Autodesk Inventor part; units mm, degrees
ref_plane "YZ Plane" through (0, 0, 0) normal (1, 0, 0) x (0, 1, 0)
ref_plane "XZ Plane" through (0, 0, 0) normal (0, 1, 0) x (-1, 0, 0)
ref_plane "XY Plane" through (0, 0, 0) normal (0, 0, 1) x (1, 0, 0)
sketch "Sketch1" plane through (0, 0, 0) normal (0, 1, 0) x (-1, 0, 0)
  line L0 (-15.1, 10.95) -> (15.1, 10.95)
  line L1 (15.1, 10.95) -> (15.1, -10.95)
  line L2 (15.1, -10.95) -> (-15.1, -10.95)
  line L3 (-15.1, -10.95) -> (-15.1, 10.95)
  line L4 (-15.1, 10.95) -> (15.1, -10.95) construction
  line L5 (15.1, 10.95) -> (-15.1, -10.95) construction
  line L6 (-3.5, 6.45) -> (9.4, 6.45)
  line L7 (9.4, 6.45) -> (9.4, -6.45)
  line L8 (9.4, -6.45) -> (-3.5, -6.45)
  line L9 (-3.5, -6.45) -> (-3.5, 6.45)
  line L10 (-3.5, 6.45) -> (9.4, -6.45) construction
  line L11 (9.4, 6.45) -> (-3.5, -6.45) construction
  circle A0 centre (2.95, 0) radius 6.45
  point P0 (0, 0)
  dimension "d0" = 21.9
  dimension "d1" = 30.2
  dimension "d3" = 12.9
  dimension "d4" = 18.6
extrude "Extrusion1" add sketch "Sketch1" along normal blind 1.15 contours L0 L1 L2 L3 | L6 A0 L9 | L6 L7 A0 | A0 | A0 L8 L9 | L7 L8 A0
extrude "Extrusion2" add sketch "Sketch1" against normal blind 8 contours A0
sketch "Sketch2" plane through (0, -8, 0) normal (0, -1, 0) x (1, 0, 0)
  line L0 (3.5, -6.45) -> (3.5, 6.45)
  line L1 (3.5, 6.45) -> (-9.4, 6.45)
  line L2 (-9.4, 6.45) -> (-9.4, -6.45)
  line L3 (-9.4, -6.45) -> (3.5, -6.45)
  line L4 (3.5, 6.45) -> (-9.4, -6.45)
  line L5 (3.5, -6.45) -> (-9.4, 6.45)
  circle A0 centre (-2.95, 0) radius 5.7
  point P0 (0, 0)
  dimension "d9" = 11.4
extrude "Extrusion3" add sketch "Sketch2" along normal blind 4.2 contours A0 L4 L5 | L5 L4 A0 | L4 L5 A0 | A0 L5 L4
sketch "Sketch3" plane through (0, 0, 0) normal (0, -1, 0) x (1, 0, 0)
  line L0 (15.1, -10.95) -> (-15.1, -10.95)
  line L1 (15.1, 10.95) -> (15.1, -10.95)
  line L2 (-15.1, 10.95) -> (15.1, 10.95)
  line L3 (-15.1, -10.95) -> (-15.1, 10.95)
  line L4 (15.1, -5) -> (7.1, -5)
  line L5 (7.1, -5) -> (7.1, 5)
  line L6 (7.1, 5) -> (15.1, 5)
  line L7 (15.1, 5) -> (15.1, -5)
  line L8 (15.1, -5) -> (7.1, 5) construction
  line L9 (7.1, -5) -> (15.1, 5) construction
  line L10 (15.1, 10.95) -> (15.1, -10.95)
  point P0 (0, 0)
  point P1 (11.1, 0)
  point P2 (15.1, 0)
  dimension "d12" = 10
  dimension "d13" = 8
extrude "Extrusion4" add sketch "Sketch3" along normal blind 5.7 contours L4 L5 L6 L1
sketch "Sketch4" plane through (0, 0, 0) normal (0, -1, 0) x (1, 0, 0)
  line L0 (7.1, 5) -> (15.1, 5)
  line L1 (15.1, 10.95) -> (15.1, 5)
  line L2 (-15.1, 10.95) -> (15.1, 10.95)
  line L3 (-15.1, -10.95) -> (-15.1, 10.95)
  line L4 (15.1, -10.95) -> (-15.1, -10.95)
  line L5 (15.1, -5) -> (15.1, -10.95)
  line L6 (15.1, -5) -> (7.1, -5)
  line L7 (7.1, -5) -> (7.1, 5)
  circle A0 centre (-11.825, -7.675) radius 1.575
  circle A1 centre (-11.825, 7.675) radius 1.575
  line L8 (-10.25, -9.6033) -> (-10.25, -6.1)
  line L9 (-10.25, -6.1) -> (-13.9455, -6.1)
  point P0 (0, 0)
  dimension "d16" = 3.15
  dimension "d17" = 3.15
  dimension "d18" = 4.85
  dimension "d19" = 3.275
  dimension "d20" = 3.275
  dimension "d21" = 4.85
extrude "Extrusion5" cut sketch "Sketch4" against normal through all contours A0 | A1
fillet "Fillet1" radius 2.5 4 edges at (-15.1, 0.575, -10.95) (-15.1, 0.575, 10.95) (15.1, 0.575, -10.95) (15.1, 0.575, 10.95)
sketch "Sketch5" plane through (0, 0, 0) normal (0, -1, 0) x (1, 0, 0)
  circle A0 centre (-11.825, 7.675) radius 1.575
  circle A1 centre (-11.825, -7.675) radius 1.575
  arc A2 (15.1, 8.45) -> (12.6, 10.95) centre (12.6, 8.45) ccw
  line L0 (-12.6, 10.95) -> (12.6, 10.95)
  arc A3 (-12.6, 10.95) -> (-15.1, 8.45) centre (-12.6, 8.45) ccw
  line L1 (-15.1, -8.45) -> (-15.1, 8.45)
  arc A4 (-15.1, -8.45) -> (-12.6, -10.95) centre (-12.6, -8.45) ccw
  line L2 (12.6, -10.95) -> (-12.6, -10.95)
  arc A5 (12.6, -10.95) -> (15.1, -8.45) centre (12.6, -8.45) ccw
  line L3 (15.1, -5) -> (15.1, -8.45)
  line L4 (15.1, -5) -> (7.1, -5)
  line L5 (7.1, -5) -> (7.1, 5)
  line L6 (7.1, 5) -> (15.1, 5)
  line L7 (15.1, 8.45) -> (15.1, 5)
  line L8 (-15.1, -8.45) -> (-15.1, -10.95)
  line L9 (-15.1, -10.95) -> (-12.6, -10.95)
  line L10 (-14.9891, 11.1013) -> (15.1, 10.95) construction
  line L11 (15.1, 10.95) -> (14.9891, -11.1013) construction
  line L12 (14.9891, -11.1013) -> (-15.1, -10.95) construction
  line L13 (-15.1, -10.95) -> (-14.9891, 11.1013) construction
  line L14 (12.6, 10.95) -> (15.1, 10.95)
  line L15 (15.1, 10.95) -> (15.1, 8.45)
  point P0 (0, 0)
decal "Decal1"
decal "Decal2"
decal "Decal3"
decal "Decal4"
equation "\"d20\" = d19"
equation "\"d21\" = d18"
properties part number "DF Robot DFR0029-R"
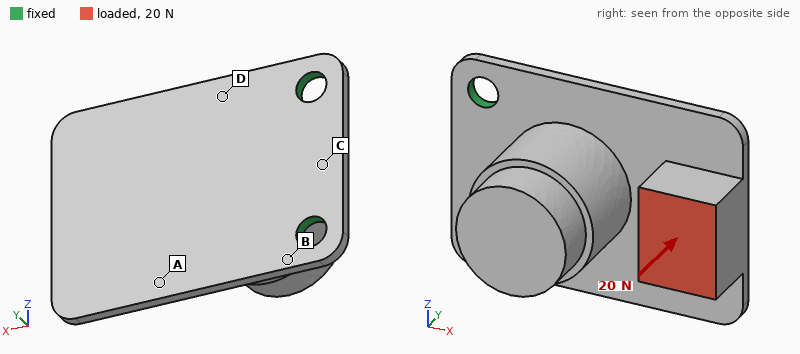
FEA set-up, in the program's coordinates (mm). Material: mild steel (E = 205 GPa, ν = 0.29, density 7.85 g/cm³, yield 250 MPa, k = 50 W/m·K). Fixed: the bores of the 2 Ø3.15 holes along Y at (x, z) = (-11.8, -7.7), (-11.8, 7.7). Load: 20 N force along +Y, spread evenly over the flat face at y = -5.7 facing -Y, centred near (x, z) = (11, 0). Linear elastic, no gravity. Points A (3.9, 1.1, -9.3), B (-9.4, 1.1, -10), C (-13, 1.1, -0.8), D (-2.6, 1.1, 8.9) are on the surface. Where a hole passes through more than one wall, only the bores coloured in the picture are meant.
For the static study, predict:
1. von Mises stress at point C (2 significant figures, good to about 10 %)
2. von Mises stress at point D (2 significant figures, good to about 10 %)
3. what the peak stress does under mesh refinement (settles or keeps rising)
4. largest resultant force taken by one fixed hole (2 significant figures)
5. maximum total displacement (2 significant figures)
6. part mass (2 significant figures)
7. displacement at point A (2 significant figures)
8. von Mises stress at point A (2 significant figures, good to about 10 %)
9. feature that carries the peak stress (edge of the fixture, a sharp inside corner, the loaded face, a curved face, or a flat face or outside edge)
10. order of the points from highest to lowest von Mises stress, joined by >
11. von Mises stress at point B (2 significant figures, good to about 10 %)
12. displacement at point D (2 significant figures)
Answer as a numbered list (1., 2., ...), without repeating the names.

1. 27 MPa
2. 8.9 MPa
3. keeps rising
4. 10 N
5. 77 µm
6. 21 g
7. 33 µm
8. 18 MPa
9. edge of the fixture
10. B > C > A > D
11. 67 MPa
12. 16 µm
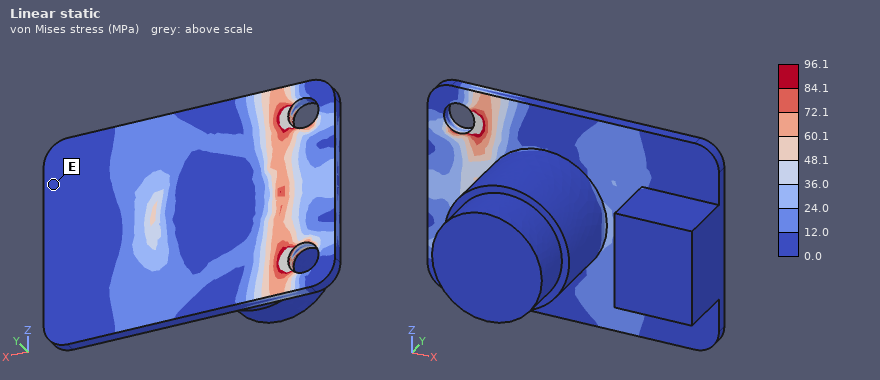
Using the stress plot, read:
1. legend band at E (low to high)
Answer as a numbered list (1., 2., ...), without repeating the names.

1. 0.0 to 12.0 MPa
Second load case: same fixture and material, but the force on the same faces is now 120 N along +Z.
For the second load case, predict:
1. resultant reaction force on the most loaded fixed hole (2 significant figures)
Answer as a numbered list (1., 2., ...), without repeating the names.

1. 190 N
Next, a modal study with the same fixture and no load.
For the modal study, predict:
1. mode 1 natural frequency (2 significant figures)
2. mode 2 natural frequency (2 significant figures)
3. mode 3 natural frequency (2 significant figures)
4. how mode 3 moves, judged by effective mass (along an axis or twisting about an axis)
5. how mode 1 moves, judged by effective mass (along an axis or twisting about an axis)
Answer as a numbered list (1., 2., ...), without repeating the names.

1. 1000 Hz
2. 4400 Hz
3. 5200 Hz
4. along Z
5. along Y
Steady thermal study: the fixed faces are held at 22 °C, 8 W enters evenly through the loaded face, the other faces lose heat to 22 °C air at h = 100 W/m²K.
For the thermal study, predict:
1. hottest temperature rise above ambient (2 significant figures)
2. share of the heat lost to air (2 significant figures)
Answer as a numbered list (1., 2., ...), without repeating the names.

1. 67 K
2. 65 %
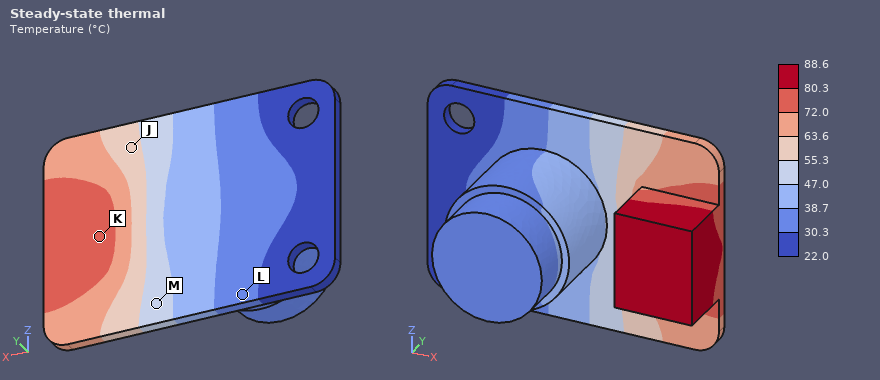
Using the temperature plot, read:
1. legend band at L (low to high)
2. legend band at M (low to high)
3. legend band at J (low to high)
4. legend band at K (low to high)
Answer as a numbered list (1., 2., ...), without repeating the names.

1. 30.3 to 38.7 °C
2. 47.0 to 55.3 °C
3. 55.3 to 63.6 °C
4. 72.0 to 80.3 °C
